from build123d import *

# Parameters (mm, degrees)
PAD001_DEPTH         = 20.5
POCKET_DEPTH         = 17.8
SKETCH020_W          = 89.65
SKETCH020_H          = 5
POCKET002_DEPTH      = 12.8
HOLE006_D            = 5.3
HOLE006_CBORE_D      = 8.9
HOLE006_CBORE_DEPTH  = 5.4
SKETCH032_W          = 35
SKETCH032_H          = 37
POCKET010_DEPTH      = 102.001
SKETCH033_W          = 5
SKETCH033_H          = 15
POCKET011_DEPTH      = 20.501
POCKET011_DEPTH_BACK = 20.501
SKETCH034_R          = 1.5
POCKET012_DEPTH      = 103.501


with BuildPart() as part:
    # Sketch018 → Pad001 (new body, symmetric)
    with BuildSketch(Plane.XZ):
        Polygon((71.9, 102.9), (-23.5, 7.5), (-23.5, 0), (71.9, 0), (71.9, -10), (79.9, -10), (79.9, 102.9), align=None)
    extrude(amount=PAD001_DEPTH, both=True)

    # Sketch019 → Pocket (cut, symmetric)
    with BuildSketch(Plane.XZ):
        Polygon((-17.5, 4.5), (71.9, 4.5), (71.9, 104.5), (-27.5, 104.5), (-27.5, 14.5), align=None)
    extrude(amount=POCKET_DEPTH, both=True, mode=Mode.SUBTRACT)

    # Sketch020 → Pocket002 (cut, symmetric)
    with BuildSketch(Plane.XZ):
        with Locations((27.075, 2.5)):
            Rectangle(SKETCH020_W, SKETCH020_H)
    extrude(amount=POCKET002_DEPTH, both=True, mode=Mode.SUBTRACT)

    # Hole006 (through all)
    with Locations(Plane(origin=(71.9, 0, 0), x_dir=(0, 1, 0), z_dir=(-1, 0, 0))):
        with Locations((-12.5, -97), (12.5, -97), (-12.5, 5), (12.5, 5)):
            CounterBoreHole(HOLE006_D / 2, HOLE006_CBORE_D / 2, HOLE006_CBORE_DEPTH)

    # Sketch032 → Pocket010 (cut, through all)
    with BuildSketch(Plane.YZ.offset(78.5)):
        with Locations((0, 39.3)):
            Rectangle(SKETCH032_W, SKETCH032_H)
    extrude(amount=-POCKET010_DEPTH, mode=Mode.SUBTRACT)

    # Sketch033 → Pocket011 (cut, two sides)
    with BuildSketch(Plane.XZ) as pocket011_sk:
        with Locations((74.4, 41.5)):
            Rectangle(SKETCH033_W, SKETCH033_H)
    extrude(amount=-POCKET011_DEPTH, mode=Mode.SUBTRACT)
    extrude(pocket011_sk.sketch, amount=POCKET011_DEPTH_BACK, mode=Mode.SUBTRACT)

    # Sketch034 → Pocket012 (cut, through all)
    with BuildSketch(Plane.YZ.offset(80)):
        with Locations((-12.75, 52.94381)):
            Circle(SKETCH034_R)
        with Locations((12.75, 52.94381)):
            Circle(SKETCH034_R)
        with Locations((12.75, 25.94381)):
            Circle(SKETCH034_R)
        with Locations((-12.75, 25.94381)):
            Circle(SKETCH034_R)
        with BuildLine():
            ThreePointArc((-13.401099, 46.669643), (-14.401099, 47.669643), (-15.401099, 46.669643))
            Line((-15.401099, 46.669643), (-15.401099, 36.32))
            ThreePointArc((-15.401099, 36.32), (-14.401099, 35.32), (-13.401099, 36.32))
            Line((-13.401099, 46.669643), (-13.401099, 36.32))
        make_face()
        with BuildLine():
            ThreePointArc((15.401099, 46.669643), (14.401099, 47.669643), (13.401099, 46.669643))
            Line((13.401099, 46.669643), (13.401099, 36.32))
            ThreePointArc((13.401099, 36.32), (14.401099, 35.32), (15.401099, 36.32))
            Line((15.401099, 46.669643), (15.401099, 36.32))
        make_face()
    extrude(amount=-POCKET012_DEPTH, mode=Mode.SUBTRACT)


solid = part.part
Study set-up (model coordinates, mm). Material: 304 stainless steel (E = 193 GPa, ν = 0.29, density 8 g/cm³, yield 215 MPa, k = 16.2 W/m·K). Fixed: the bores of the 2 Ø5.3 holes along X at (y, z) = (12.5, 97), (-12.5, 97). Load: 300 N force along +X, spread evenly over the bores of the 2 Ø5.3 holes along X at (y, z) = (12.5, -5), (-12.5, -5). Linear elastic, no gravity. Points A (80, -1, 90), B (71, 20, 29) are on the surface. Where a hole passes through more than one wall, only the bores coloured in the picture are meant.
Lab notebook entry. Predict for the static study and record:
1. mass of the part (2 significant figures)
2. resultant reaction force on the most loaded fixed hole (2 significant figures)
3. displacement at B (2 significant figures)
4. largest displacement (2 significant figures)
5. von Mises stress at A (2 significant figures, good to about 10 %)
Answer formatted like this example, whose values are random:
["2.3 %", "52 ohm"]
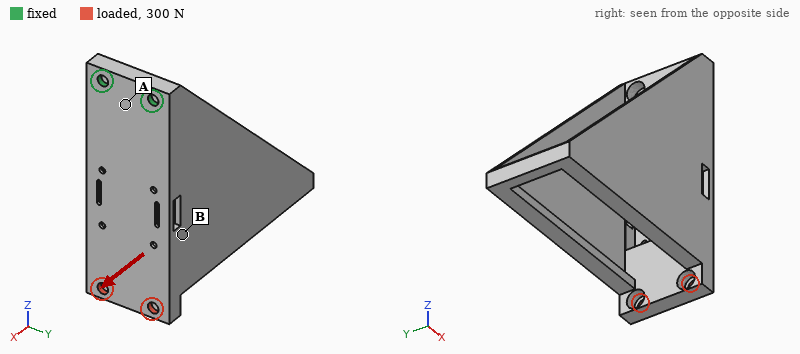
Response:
["480 g", "360 N", "0.18 mm", "0.38 mm", "37 MPa"]
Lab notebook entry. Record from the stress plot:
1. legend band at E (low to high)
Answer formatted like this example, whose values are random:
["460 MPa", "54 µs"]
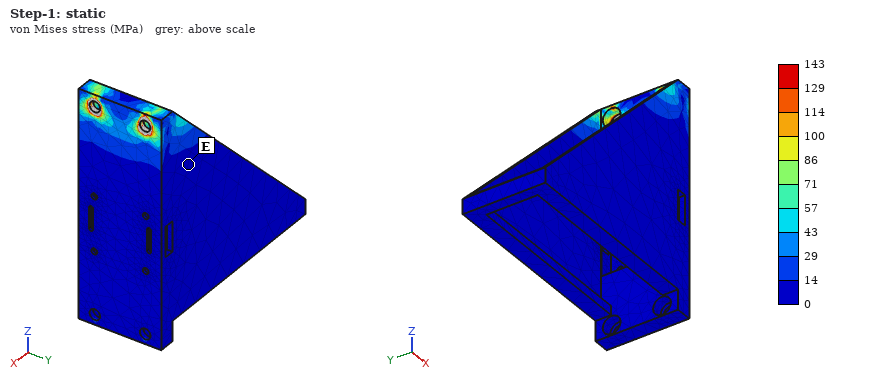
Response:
["0 to 14 MPa"]
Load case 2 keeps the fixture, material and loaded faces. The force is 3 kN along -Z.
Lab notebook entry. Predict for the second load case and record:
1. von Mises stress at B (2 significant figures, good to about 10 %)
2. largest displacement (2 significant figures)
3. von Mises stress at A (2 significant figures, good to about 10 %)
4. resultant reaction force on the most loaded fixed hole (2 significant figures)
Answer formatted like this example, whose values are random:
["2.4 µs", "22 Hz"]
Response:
["17 MPa", "38 µm", "12 MPa", "1.5 kN"]
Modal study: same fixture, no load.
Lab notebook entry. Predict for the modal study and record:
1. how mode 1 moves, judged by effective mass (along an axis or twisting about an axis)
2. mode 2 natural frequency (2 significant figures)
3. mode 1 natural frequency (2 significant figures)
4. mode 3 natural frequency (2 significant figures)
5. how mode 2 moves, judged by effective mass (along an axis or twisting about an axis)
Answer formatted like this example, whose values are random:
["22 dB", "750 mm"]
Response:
["along X", "350 Hz", "320 Hz", "1300 Hz", "along Y"]
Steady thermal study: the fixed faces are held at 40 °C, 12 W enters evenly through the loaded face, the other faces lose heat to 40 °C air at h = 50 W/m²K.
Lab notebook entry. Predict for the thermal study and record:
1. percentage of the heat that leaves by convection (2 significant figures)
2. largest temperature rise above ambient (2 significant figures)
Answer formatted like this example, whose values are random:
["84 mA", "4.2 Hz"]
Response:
["99 %", "75 K"]
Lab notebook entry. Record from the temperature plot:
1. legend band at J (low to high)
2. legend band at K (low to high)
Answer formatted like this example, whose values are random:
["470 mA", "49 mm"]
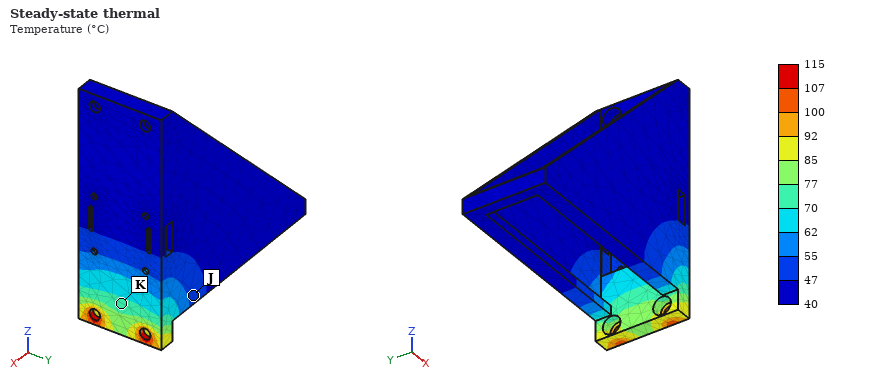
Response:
["47 to 55 °C", "70 to 77 °C"]
